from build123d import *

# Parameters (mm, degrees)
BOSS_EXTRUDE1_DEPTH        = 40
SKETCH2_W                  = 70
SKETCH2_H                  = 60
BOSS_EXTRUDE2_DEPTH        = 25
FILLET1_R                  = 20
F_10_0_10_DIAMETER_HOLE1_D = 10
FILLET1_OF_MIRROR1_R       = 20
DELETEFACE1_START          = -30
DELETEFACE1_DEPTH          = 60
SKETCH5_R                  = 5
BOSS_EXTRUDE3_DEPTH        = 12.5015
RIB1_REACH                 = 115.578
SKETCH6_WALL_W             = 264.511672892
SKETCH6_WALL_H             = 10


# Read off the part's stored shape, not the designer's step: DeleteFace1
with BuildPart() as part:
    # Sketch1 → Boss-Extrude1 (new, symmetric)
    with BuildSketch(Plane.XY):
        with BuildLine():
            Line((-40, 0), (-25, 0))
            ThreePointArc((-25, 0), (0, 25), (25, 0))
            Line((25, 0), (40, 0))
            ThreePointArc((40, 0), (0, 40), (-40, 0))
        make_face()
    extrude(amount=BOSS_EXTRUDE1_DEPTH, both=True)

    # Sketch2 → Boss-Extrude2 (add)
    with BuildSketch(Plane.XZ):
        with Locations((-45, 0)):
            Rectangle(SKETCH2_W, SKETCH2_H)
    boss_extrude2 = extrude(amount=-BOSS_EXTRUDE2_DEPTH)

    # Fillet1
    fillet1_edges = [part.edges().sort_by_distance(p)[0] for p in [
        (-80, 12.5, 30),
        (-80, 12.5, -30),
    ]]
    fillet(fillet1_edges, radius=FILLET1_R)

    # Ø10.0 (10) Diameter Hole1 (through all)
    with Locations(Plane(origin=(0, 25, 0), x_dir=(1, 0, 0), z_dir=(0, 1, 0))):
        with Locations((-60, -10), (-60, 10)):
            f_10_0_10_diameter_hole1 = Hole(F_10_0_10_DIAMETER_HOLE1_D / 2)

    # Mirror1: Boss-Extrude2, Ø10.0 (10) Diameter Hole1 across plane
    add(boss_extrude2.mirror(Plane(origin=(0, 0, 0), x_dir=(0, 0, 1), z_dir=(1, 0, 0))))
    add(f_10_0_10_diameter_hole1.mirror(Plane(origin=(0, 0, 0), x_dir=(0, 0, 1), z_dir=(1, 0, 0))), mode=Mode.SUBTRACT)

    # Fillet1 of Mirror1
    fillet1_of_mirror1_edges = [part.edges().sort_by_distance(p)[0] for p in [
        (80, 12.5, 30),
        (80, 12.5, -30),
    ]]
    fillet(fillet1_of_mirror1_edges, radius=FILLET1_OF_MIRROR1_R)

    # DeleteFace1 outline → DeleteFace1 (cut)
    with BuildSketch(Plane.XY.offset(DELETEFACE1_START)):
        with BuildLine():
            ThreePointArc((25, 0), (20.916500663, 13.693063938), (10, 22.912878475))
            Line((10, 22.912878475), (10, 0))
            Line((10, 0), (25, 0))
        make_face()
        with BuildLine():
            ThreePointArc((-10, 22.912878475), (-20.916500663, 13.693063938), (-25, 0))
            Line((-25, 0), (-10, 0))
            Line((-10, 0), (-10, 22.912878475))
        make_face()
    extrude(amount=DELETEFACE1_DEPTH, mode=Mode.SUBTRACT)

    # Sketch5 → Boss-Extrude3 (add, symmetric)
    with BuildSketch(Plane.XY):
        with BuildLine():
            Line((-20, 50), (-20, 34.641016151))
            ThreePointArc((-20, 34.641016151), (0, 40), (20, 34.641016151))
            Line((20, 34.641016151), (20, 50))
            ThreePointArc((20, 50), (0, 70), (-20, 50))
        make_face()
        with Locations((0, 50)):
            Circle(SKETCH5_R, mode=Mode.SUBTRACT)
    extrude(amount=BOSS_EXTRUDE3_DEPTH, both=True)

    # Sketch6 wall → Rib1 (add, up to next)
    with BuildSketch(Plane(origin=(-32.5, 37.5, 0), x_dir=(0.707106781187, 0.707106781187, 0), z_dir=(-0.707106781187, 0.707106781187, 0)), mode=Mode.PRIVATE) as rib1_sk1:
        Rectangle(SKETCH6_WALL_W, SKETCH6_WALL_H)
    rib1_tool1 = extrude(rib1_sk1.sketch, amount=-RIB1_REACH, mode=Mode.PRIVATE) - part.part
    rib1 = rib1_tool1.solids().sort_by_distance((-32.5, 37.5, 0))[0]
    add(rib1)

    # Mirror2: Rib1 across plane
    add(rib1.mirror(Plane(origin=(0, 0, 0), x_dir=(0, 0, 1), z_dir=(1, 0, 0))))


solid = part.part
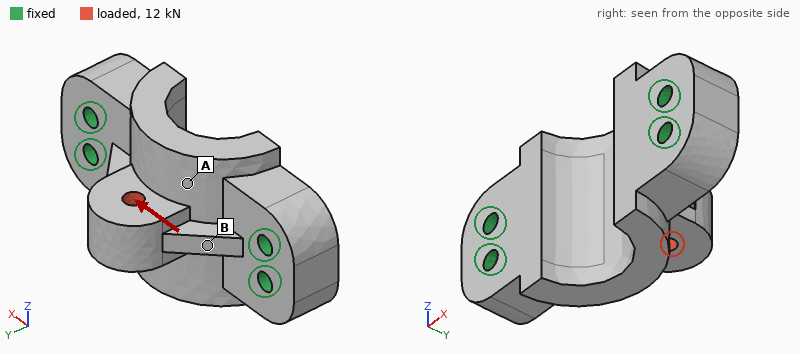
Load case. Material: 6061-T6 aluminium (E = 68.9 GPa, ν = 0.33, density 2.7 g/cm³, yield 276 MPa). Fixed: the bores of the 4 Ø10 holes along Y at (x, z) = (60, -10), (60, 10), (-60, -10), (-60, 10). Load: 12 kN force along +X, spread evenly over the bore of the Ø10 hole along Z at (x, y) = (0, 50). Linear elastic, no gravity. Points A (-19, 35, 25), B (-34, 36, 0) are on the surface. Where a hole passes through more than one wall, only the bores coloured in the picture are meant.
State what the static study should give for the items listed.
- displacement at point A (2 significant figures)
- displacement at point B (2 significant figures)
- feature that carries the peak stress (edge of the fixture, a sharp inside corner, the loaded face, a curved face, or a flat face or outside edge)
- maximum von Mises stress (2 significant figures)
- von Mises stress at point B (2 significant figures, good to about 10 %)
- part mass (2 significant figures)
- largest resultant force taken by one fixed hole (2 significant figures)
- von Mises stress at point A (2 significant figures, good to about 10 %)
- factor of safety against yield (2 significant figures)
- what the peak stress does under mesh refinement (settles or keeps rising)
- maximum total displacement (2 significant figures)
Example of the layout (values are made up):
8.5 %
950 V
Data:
6.5 µm
9.4 µm
the loaded face
39 MPa
29 MPa
720 g
3.9 kN
5.6 MPa
7.0
settles
27 µm
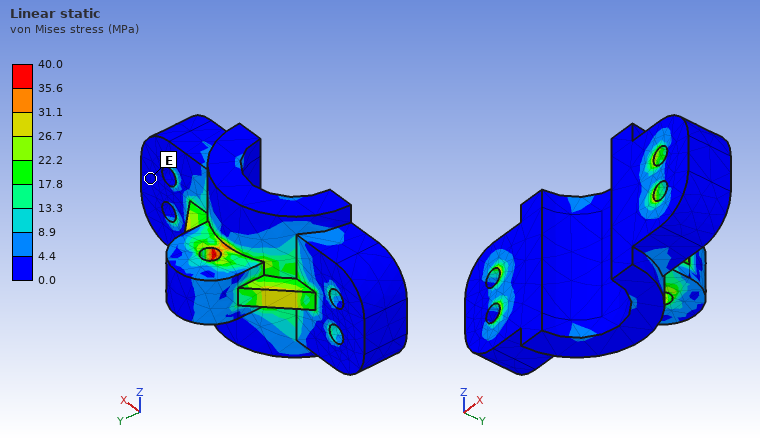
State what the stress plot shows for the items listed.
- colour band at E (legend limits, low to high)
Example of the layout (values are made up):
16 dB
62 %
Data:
0.0 to 4.4 MPa
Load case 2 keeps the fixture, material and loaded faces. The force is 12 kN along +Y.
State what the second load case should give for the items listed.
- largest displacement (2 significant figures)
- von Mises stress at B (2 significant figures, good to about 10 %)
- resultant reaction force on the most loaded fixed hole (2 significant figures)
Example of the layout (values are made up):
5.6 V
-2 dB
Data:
21 µm
18 MPa
4.4 kN
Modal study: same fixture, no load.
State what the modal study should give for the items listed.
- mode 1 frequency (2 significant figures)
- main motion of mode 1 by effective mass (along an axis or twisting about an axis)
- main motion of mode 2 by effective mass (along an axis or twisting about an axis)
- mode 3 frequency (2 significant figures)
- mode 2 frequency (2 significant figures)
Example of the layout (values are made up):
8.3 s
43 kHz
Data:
4800 Hz
along Z
along Y
10 kHz
7500 Hz
